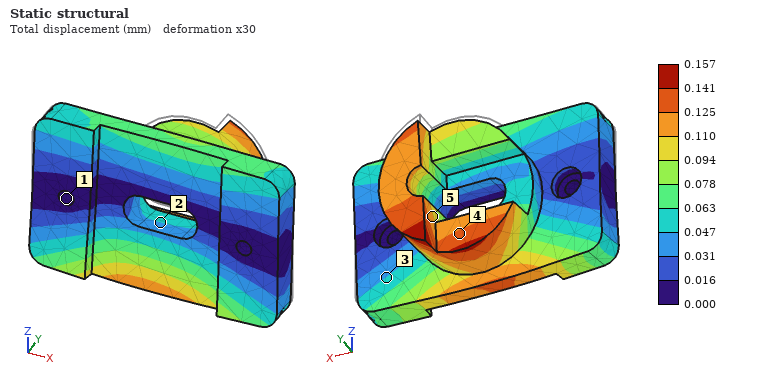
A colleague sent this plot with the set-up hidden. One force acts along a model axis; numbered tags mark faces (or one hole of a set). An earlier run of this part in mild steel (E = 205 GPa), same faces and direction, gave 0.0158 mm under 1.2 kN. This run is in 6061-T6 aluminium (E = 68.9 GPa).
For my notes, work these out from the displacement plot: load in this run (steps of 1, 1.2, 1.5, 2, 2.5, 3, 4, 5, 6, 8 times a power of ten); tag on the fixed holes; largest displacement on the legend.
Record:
4 kN
1
0.157 mm
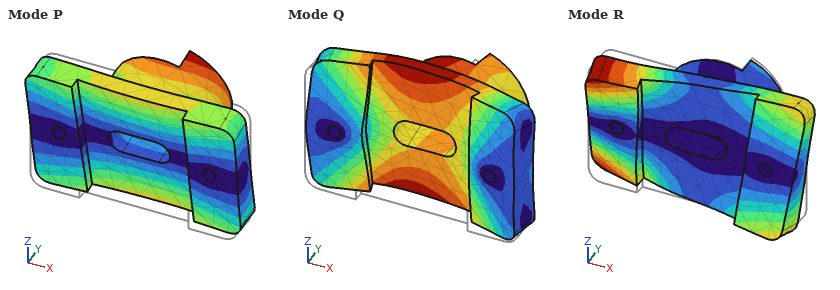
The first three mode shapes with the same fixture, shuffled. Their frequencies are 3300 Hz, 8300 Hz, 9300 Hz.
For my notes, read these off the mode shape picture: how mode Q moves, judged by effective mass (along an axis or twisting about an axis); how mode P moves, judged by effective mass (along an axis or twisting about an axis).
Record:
along Y
along Z
